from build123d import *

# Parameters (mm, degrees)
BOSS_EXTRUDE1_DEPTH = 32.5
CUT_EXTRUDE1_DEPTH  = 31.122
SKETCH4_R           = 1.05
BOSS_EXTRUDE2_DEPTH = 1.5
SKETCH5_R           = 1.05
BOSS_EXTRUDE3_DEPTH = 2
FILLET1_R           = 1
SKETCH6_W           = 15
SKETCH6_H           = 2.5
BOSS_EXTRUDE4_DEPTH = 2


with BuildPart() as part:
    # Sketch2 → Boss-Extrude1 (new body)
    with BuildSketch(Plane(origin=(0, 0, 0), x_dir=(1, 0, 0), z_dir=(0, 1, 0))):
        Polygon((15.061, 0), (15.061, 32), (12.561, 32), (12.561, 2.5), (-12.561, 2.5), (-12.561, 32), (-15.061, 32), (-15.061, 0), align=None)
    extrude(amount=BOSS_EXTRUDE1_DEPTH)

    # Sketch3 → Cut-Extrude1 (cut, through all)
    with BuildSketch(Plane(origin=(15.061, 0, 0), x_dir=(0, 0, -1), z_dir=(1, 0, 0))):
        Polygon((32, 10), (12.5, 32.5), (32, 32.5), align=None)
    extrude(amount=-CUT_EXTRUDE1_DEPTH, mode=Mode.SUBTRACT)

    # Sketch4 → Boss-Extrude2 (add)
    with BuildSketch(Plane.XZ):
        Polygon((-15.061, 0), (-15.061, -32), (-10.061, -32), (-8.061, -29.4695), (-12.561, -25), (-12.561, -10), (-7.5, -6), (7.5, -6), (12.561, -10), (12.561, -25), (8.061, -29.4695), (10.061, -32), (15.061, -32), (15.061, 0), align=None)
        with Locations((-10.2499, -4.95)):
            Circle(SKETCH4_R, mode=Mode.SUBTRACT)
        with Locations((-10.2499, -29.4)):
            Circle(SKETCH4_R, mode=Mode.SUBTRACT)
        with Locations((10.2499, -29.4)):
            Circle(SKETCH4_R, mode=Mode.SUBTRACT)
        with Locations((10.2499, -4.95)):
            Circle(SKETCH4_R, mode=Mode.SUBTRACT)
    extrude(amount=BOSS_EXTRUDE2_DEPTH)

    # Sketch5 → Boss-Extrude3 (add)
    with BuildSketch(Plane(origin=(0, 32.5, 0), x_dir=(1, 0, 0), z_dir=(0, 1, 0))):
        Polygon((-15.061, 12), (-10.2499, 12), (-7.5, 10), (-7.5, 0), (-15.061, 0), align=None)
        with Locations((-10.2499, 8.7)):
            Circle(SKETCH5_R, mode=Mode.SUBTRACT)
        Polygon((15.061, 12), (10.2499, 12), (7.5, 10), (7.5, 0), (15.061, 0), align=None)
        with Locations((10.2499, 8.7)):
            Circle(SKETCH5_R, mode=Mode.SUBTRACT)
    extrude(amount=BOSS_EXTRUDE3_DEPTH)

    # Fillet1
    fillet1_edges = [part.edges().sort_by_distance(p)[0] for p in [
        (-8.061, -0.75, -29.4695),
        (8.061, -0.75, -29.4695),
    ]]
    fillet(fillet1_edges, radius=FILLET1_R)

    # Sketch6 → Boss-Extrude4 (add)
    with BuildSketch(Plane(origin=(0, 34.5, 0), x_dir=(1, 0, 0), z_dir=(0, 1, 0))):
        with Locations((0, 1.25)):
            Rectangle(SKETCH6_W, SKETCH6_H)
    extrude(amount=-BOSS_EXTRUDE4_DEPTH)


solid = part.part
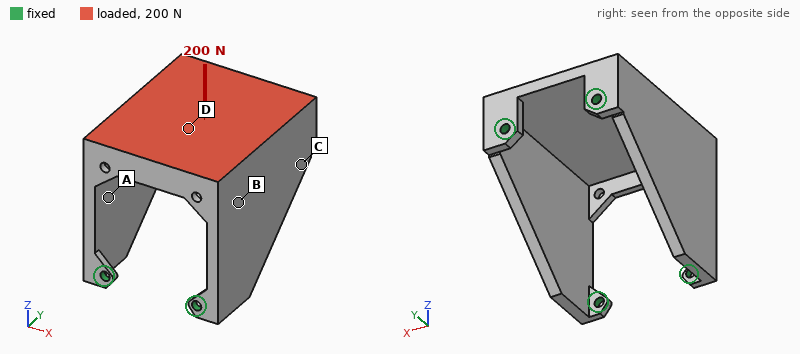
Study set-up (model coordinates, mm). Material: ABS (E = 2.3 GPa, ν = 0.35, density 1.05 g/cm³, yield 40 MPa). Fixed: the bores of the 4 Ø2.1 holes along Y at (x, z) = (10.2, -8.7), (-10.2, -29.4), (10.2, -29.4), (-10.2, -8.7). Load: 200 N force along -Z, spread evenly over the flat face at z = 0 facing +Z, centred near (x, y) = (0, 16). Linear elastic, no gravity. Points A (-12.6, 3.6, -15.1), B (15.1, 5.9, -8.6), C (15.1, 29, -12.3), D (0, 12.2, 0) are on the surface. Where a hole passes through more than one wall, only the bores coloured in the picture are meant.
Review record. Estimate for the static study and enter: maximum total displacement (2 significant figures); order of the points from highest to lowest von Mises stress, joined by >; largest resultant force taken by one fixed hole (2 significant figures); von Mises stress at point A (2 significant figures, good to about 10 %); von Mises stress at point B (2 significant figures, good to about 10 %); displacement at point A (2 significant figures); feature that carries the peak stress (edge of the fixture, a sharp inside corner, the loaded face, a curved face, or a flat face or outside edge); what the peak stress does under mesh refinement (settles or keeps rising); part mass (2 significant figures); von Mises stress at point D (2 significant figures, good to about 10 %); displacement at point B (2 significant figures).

0.21 mm
D > A > B > C
55 N
4.5 MPa
2.4 MPa
0.11 mm
edge of the fixture
keeps rising
7.4 g
6.6 MPa
0.087 mm
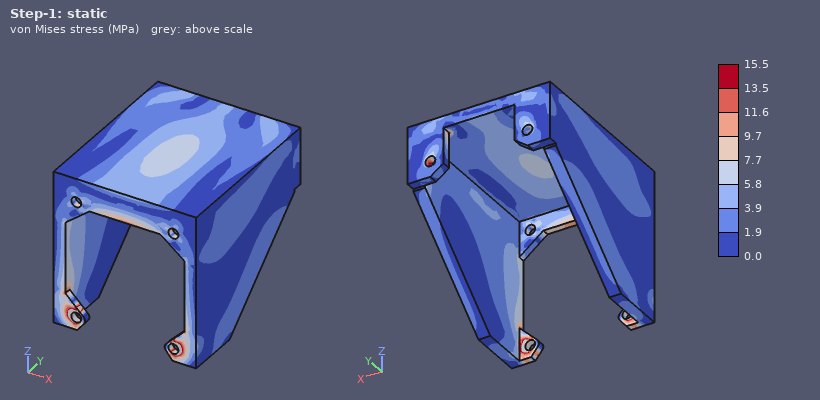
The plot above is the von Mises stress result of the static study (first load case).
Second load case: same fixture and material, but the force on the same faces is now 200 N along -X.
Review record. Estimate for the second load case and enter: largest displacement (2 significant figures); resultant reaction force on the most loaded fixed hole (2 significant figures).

0.54 mm
140 N
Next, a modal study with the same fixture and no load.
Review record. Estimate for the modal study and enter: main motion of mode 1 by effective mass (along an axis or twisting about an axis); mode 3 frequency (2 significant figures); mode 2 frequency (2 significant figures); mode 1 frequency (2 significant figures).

along X
2200 Hz
2100 Hz
1600 Hz
